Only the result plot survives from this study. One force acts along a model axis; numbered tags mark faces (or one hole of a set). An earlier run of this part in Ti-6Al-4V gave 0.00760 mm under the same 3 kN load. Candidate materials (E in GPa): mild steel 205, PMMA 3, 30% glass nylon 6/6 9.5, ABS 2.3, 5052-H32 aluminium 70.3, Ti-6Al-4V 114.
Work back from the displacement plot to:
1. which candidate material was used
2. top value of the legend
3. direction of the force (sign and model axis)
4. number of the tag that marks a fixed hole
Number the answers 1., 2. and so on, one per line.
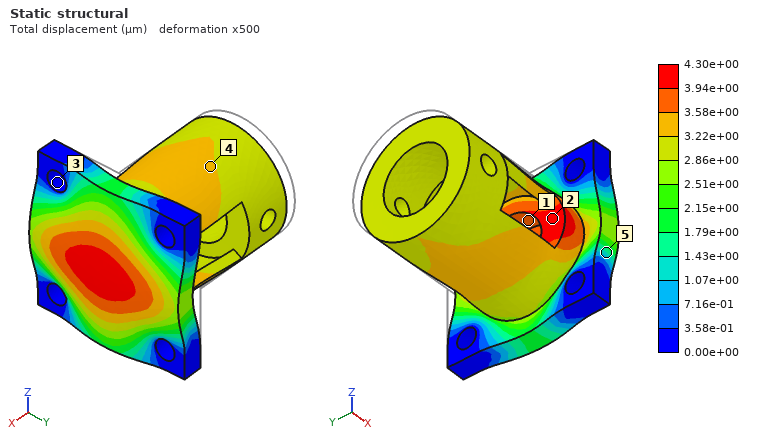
1. mild steel
2. 4.30e+00 µm
3. +X
4. 3
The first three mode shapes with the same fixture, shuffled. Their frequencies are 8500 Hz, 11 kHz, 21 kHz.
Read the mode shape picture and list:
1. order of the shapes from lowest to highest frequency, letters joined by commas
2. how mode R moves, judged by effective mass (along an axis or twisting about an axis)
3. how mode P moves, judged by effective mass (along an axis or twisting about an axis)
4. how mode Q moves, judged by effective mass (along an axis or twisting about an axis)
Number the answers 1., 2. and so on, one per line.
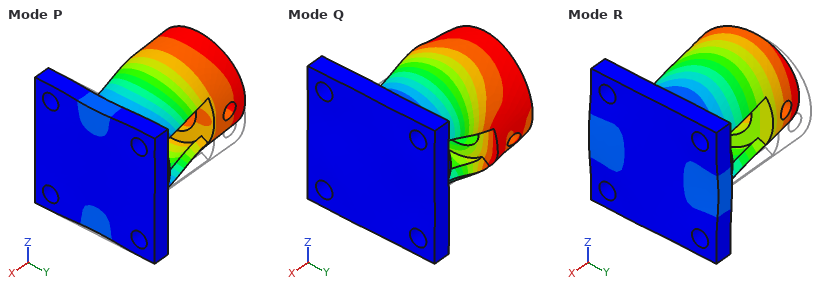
1. P, R, Q
2. along Y
3. along Z
4. twisting about X
